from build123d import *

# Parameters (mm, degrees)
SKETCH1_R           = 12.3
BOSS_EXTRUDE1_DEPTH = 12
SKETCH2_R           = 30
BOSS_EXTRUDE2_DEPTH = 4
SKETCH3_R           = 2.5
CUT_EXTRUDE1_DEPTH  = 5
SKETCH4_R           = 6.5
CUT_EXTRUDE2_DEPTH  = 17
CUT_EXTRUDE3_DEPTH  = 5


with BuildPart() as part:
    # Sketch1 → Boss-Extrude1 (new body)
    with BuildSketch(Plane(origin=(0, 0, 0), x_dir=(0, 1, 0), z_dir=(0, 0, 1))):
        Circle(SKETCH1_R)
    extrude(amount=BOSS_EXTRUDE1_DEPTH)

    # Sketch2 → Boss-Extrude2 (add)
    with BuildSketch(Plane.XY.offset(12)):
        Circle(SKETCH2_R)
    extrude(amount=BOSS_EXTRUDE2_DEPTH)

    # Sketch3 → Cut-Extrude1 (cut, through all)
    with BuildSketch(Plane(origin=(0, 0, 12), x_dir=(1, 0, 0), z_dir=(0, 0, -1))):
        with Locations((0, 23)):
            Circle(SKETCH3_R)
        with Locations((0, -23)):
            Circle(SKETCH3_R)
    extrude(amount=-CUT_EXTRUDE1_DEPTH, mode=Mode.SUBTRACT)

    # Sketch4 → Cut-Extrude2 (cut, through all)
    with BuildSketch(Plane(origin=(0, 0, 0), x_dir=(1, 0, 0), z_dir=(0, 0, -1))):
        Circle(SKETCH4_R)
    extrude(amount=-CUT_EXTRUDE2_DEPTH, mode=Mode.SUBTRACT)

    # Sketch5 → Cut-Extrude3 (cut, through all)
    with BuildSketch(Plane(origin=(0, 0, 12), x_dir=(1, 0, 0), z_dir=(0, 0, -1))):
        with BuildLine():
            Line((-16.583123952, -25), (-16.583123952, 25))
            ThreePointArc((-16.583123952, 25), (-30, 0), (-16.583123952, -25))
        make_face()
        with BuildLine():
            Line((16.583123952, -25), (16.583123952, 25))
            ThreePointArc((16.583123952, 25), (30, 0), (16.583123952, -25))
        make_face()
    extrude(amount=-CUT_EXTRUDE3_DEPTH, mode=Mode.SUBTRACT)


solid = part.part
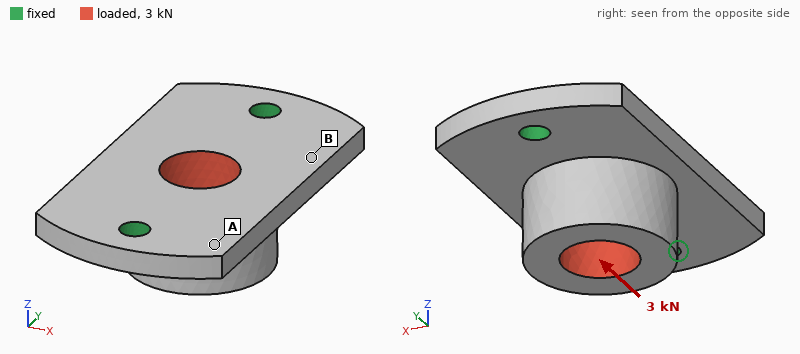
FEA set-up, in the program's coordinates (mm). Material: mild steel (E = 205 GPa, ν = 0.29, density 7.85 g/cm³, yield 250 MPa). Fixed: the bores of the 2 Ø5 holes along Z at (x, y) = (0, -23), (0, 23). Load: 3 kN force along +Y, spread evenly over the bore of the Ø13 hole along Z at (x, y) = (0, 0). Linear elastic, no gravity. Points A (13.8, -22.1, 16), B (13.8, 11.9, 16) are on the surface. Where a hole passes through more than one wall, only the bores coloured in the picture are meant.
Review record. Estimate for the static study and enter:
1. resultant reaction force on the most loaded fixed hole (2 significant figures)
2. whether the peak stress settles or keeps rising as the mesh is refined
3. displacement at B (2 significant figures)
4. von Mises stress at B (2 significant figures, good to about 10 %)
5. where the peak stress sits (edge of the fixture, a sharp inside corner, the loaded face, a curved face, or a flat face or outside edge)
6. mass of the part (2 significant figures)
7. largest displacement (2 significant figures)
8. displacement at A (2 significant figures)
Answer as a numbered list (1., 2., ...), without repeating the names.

1. 1.6 kN
2. keeps rising
3. 2.8 µm
4. 13 MPa
5. edge of the fixture
6. 86 g
7. 7.3 µm
8. 2.1 µm
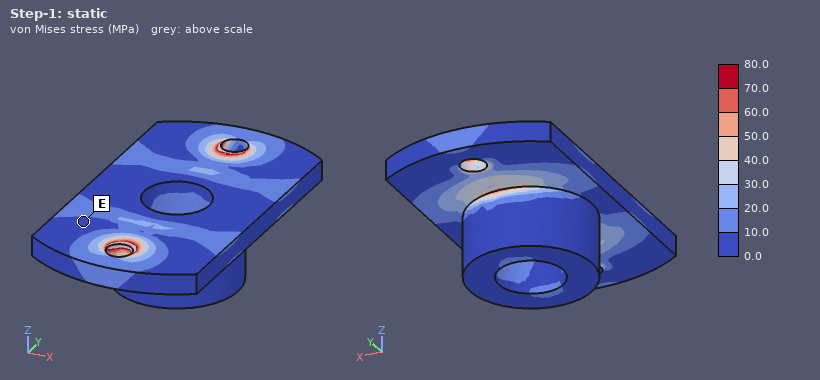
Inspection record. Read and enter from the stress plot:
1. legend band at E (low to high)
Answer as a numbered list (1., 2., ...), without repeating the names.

1. 0.0 to 10.0 MPa
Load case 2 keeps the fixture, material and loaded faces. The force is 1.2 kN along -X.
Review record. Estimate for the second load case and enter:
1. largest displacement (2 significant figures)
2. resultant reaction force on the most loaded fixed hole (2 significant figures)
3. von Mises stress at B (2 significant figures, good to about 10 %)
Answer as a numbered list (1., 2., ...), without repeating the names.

1. 18 µm
2. 600 N
3. 19 MPa
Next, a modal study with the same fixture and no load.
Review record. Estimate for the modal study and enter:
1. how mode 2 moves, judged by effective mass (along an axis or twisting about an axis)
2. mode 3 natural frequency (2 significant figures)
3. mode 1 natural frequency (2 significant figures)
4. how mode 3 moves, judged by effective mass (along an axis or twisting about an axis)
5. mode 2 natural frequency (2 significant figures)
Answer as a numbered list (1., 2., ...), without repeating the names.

1. along Z
2. 14 kHz
3. 5300 Hz
4. along Y
5. 8500 Hz
